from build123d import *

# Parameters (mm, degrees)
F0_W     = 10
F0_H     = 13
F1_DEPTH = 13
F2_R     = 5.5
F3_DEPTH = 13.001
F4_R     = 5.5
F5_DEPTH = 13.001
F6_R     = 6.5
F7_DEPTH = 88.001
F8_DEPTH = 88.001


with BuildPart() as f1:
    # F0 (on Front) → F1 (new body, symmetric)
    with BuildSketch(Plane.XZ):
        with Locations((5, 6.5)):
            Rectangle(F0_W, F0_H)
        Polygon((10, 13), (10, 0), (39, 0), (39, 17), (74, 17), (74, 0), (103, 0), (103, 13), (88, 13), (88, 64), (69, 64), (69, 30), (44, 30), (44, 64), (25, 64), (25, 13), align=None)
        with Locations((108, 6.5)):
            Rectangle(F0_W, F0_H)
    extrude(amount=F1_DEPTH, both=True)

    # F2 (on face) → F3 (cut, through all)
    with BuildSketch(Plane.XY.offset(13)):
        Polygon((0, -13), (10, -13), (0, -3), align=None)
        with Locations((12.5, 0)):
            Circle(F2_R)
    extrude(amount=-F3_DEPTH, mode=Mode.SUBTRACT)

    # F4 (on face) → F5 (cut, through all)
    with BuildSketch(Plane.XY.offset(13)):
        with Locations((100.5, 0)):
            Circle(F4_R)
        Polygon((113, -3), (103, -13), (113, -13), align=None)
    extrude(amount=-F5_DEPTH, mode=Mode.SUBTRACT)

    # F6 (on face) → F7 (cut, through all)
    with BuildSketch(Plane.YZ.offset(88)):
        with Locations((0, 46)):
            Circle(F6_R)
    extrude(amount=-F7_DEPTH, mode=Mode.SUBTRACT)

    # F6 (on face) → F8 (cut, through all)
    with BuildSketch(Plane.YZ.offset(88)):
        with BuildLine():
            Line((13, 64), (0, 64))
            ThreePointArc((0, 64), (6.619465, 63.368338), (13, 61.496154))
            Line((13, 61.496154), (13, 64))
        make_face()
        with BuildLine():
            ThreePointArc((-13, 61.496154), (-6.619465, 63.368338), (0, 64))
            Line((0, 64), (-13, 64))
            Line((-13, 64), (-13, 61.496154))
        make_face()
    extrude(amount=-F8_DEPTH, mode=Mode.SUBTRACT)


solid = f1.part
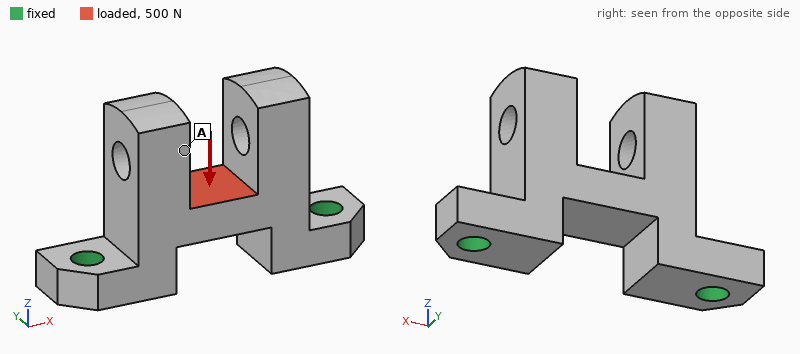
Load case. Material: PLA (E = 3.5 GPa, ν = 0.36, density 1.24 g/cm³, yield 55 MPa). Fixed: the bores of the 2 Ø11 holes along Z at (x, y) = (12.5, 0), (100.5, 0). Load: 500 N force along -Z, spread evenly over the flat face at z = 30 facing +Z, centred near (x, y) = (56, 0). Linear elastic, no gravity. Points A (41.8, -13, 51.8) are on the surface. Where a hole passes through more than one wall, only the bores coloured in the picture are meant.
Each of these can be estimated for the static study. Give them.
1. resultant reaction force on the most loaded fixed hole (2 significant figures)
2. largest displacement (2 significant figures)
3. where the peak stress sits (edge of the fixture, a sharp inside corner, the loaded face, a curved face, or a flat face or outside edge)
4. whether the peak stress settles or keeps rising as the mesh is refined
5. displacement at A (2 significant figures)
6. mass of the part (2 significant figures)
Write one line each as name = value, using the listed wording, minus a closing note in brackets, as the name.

resultant reaction force on the most loaded fixed hole = 370 N
largest displacement = 55 µm
where the peak stress sits = edge of the fixture
whether the peak stress settles or keeps rising as the mesh is refined = keeps rising
displacement at A = 43 µm
mass of the part = 92 g
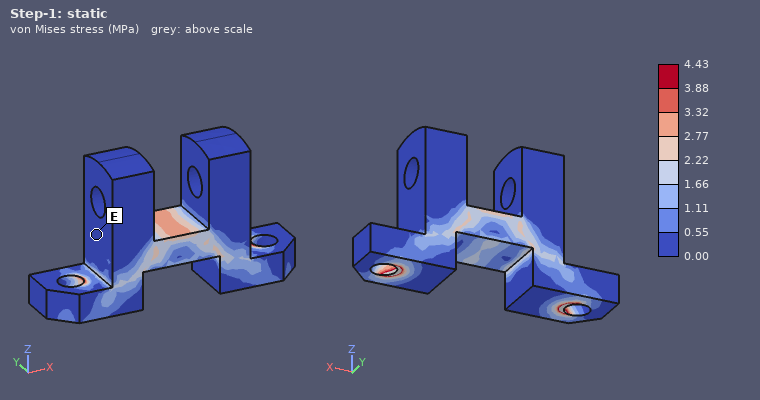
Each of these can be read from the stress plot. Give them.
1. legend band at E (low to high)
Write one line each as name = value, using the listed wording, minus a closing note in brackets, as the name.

legend band at E = 0.00 to 0.55 MPa
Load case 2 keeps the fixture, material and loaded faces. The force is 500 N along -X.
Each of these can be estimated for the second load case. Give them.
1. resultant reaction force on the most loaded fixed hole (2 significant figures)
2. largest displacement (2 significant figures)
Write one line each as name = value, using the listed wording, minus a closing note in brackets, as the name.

resultant reaction force on the most loaded fixed hole = 290 N
largest displacement = 30 µm
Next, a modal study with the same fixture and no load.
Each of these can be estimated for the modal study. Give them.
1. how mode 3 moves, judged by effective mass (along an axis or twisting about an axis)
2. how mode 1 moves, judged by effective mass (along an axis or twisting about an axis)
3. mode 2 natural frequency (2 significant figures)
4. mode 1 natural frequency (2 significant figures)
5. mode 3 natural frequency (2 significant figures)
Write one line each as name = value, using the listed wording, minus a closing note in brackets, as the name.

how mode 3 moves, judged by effective mass = along X
how mode 1 moves, judged by effective mass = along Y
mode 2 natural frequency = 1400 Hz
mode 1 natural frequency = 890 Hz
mode 3 natural frequency = 1900 Hz
